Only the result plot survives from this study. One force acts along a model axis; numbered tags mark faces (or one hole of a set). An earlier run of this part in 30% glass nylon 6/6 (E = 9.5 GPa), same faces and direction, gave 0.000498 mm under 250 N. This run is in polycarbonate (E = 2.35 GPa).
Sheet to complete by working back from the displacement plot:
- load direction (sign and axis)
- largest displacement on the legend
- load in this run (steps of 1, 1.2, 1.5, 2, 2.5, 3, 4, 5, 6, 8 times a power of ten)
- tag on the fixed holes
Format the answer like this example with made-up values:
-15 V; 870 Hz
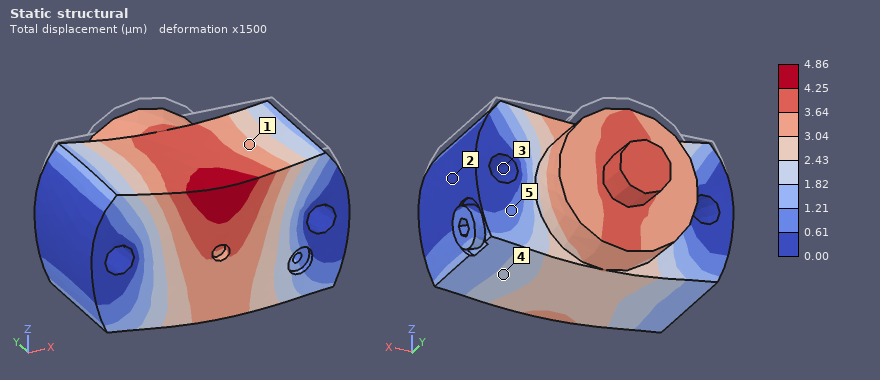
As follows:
-Z; 4.86 µm; 600 N; 3
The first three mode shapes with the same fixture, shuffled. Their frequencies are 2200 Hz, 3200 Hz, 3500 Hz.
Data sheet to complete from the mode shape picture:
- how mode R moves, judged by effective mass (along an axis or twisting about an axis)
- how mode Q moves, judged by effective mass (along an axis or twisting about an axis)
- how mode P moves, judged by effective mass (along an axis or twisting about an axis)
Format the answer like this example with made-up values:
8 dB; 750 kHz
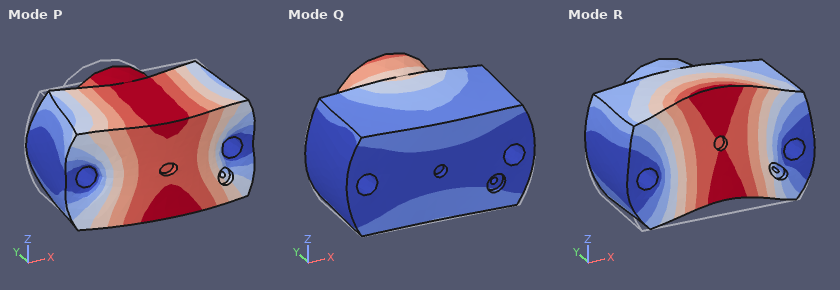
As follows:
along Z; along Z; along Y
